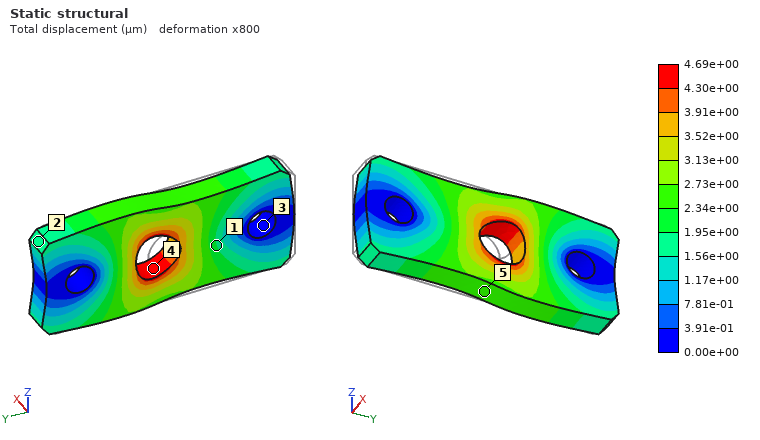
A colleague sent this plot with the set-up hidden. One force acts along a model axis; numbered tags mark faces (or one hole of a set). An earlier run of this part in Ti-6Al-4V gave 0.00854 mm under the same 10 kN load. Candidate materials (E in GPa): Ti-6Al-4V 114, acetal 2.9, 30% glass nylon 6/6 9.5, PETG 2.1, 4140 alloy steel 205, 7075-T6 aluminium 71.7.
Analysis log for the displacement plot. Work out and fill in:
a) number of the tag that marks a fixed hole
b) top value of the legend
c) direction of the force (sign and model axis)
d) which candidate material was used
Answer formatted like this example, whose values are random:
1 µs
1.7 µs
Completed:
3
4.69e+00 µm
+Y
4140 alloy steel
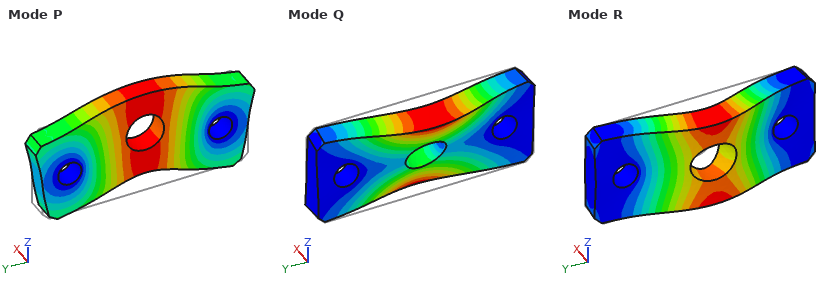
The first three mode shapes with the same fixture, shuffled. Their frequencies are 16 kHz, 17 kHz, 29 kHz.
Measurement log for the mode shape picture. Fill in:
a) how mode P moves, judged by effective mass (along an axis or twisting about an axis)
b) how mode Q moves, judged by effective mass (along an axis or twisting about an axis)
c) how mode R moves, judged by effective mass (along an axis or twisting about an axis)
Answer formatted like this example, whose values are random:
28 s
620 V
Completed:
along Z
twisting about Y
along X
